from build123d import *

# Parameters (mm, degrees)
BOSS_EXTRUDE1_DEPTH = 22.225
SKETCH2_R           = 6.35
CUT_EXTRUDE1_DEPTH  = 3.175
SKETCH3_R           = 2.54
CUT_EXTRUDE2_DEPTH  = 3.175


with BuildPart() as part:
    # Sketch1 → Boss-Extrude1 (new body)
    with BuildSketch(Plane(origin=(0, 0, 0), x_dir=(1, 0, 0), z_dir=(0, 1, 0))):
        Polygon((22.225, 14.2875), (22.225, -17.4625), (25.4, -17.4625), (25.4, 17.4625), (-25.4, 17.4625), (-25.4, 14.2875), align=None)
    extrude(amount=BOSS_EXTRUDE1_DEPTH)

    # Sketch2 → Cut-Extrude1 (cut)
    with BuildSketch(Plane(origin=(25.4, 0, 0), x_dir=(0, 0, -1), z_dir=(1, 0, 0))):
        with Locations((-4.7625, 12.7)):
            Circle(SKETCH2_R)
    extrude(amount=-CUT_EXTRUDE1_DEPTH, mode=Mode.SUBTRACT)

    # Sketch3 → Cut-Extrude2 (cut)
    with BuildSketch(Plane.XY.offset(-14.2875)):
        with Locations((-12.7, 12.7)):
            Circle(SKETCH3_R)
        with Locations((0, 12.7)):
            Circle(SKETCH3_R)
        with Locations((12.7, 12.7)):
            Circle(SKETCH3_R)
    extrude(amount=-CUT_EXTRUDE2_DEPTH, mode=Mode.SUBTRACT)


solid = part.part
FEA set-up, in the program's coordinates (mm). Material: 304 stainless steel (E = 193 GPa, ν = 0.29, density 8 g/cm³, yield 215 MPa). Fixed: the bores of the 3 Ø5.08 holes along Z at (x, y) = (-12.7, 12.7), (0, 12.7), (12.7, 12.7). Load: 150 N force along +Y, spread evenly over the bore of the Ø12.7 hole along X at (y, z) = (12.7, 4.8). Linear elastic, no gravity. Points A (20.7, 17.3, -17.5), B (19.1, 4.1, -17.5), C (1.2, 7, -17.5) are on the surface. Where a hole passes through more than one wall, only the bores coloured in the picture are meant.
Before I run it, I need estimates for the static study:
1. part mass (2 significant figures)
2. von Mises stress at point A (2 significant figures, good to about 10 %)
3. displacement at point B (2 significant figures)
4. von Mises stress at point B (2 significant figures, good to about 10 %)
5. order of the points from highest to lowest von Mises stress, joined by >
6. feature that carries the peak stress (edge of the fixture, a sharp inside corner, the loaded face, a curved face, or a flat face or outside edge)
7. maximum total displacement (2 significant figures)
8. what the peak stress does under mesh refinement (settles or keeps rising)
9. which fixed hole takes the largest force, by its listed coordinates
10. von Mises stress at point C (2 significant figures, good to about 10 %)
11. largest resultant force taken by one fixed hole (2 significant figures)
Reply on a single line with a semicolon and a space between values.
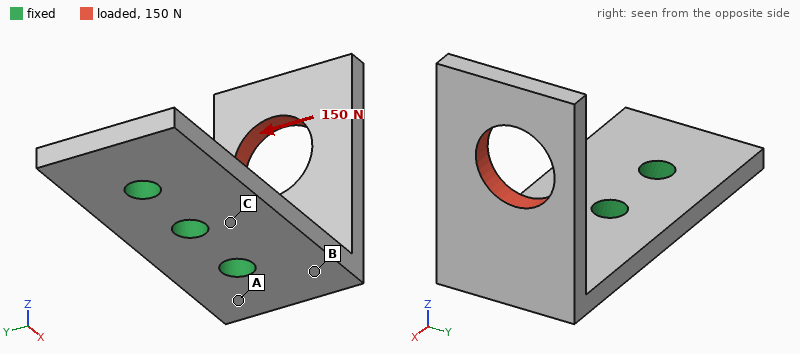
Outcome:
42 g; 38 MPa; 8.5 µm; 24 MPa; A > B > C; edge of the fixture; 55 µm; keeps rising; (12.7, 12.7); 10 MPa; 210 N
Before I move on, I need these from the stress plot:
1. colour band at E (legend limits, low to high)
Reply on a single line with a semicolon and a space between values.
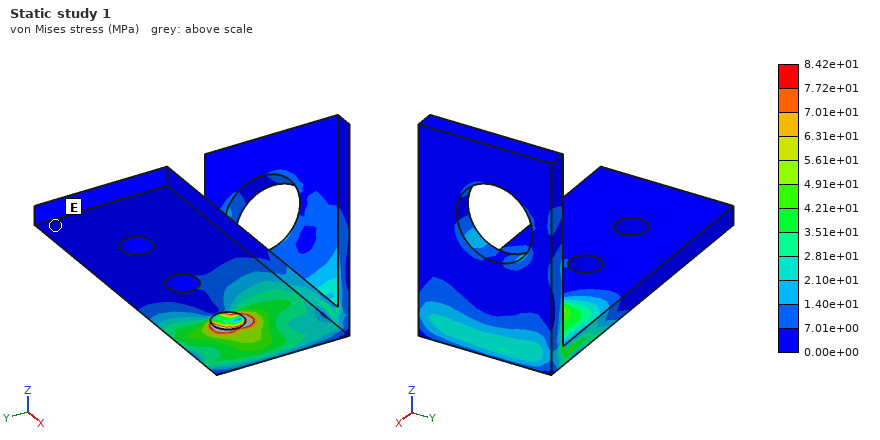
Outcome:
0.00e+00 to 7.01e+00 MPa
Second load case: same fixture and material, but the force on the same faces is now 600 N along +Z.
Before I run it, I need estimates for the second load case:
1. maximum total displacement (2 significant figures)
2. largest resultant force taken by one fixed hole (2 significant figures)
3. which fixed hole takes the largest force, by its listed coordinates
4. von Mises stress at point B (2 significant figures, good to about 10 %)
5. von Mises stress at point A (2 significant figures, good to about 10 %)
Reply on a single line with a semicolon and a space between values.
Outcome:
98 µm; 700 N; (12.7, 12.7); 56 MPa; 48 MPa
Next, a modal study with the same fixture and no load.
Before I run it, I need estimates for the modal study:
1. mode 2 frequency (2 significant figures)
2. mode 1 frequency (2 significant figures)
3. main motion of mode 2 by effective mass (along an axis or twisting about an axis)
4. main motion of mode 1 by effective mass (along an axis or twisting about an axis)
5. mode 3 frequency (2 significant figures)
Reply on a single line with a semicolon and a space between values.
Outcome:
2800 Hz; 1700 Hz; along Y; along X; 6200 Hz
